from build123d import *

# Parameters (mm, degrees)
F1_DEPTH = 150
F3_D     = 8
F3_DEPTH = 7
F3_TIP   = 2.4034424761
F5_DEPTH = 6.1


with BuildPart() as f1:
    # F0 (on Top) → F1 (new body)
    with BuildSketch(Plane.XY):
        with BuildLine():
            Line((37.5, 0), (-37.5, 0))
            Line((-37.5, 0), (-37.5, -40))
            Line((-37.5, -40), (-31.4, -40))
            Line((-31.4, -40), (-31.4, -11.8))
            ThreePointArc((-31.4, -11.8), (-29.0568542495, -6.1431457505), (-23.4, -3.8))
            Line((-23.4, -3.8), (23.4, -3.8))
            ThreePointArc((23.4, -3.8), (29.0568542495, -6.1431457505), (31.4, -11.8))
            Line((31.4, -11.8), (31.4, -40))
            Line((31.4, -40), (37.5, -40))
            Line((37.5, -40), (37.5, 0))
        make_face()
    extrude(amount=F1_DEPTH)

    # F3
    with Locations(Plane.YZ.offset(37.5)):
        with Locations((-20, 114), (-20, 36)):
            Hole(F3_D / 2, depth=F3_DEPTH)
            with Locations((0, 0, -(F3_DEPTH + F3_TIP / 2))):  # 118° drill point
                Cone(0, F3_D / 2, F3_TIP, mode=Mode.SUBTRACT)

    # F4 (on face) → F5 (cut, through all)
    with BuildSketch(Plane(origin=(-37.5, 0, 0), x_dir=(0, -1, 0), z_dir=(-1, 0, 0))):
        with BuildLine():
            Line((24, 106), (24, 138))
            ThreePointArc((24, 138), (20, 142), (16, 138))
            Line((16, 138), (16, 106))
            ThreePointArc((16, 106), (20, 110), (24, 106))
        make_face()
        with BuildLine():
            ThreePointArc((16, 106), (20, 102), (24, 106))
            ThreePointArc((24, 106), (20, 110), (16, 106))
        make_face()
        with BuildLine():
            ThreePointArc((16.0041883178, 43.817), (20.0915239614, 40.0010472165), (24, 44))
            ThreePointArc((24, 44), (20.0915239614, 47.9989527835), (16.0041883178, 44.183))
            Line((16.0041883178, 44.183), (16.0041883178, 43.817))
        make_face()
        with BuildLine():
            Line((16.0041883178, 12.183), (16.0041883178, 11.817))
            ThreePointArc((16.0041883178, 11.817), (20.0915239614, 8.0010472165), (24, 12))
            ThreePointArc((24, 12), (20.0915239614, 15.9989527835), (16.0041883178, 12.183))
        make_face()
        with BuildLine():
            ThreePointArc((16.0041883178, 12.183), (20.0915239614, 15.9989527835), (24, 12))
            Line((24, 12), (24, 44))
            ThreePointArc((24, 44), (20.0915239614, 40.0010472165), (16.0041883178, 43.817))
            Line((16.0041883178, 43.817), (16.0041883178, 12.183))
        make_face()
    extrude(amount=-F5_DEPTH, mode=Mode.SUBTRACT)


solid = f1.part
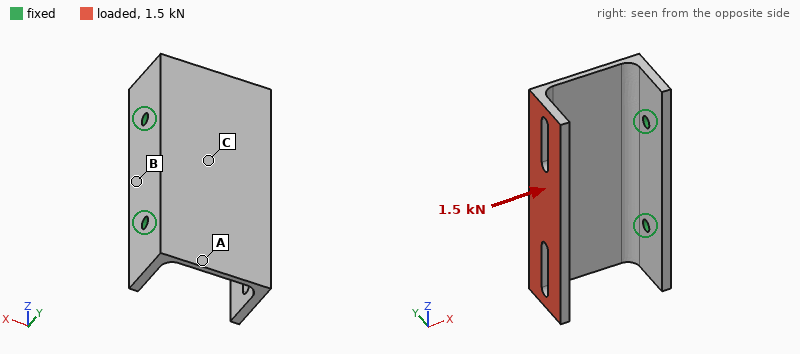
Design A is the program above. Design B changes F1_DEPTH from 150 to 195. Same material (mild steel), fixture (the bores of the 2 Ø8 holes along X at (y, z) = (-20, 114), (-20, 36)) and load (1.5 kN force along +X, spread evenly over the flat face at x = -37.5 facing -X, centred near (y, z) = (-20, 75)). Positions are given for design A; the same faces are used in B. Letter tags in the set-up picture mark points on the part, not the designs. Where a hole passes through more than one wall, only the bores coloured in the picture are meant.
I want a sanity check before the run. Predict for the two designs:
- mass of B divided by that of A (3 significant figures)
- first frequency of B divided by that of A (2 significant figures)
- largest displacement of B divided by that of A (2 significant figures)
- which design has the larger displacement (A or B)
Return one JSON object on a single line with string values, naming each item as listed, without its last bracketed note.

{"mass of B divided by that of A": "1.31", "first frequency of B divided by that of A": "0.95", "largest displacement of B divided by that of A": "0.81", "which design has the larger displacement": "A"}
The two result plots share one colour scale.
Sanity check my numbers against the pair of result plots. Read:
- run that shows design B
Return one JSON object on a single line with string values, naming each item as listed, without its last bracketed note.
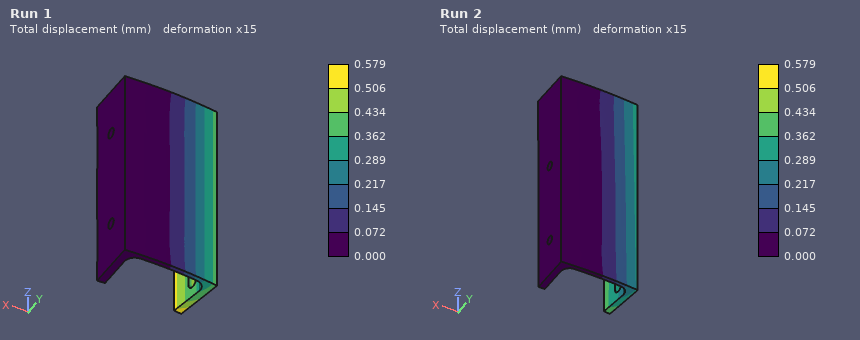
{"run that shows design B": "Run 2"}
